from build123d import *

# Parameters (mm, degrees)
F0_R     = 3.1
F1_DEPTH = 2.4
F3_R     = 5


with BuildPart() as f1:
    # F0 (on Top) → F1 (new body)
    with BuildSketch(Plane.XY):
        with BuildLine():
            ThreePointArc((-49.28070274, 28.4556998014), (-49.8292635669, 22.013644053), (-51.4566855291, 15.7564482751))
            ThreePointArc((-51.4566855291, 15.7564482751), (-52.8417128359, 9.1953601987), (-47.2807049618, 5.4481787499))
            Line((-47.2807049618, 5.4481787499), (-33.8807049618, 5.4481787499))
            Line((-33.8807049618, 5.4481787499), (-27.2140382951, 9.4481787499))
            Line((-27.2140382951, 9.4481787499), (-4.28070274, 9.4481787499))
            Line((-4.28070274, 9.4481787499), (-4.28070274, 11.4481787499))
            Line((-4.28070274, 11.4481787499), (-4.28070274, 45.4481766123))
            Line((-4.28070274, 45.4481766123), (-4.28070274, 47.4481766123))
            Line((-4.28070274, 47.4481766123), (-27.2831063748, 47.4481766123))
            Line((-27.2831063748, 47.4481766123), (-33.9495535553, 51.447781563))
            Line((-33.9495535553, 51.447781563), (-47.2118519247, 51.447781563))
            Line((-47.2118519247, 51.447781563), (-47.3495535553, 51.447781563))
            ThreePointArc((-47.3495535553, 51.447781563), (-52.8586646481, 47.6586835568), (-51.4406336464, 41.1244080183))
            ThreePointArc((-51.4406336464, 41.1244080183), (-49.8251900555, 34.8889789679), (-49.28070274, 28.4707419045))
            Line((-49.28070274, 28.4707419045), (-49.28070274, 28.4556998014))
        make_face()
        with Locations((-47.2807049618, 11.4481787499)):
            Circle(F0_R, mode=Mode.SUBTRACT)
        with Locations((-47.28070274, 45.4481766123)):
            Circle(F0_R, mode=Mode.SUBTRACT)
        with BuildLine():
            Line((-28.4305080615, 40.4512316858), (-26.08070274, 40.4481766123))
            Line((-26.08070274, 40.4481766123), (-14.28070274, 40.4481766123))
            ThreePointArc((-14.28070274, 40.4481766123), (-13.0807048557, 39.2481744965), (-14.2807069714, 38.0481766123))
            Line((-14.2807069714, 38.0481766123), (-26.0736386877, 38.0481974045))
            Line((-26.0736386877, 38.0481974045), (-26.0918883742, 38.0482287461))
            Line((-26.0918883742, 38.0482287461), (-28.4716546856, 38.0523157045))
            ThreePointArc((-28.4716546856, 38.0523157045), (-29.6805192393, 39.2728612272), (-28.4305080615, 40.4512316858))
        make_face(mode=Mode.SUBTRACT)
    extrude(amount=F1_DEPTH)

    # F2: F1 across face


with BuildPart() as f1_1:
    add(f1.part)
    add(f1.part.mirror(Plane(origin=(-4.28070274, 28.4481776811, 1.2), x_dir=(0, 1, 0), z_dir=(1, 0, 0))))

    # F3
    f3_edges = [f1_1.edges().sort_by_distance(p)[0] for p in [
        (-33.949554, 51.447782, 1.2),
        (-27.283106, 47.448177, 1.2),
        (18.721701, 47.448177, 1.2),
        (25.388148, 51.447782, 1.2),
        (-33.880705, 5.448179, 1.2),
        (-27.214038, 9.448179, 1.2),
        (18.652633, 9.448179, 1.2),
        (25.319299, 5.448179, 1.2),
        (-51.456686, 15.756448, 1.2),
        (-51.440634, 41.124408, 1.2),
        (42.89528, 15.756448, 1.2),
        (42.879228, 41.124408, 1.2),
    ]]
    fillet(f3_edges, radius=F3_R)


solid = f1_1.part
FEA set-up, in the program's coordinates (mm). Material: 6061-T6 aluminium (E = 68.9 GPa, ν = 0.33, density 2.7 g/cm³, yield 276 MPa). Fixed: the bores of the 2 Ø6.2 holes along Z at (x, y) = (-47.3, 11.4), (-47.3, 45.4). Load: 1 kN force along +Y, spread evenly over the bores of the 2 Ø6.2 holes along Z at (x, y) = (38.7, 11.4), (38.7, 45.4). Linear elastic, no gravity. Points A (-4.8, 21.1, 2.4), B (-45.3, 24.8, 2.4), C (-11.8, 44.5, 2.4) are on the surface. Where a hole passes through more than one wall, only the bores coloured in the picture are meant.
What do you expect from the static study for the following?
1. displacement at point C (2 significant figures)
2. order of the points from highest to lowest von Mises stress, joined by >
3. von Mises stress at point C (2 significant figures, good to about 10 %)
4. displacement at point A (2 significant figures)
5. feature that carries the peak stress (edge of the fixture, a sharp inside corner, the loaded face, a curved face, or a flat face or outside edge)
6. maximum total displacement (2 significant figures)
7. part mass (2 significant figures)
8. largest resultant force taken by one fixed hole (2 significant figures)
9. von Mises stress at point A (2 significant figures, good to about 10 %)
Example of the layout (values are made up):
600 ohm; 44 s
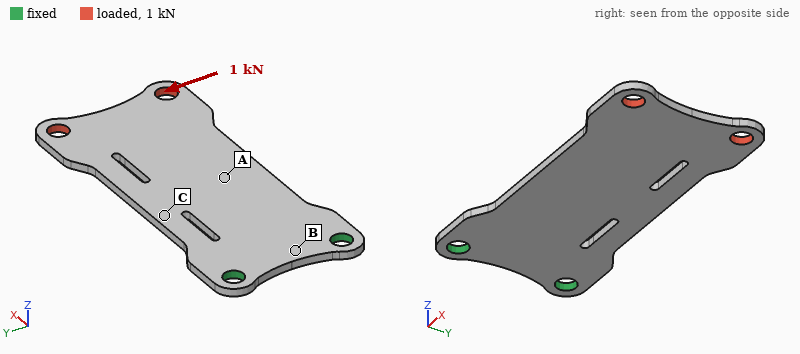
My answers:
0.074 mm; C > A > B; 83 MPa; 0.083 mm; a curved face; 0.32 mm; 24 g; 2.5 kN; 35 MPa
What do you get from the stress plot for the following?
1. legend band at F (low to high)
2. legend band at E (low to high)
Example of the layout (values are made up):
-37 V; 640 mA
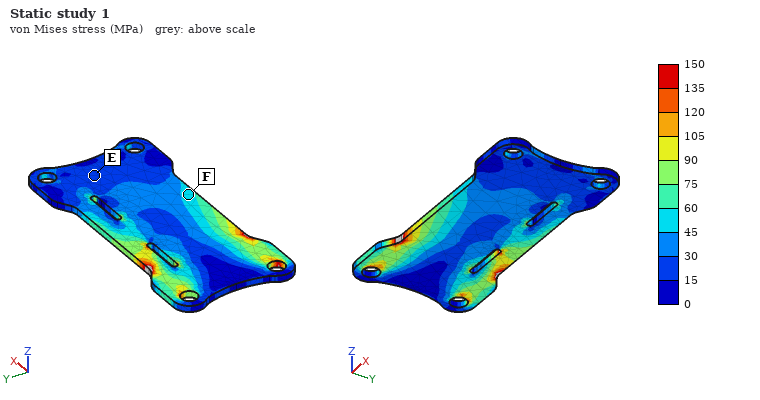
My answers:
45 to 60 MPa; 15 to 30 MPa
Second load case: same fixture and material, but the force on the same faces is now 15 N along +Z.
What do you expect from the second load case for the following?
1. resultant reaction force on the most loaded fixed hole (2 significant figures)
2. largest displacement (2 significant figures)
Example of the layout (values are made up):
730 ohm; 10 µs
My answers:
7.6 N; 1.1 mm
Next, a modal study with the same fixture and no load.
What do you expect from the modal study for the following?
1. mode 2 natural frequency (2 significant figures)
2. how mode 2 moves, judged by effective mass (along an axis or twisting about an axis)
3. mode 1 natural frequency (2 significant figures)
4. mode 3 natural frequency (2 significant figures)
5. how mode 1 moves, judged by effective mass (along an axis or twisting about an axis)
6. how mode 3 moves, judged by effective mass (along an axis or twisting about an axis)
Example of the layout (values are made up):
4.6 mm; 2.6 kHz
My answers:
1100 Hz; twisting about X; 250 Hz; 1600 Hz; along Z; along Z
